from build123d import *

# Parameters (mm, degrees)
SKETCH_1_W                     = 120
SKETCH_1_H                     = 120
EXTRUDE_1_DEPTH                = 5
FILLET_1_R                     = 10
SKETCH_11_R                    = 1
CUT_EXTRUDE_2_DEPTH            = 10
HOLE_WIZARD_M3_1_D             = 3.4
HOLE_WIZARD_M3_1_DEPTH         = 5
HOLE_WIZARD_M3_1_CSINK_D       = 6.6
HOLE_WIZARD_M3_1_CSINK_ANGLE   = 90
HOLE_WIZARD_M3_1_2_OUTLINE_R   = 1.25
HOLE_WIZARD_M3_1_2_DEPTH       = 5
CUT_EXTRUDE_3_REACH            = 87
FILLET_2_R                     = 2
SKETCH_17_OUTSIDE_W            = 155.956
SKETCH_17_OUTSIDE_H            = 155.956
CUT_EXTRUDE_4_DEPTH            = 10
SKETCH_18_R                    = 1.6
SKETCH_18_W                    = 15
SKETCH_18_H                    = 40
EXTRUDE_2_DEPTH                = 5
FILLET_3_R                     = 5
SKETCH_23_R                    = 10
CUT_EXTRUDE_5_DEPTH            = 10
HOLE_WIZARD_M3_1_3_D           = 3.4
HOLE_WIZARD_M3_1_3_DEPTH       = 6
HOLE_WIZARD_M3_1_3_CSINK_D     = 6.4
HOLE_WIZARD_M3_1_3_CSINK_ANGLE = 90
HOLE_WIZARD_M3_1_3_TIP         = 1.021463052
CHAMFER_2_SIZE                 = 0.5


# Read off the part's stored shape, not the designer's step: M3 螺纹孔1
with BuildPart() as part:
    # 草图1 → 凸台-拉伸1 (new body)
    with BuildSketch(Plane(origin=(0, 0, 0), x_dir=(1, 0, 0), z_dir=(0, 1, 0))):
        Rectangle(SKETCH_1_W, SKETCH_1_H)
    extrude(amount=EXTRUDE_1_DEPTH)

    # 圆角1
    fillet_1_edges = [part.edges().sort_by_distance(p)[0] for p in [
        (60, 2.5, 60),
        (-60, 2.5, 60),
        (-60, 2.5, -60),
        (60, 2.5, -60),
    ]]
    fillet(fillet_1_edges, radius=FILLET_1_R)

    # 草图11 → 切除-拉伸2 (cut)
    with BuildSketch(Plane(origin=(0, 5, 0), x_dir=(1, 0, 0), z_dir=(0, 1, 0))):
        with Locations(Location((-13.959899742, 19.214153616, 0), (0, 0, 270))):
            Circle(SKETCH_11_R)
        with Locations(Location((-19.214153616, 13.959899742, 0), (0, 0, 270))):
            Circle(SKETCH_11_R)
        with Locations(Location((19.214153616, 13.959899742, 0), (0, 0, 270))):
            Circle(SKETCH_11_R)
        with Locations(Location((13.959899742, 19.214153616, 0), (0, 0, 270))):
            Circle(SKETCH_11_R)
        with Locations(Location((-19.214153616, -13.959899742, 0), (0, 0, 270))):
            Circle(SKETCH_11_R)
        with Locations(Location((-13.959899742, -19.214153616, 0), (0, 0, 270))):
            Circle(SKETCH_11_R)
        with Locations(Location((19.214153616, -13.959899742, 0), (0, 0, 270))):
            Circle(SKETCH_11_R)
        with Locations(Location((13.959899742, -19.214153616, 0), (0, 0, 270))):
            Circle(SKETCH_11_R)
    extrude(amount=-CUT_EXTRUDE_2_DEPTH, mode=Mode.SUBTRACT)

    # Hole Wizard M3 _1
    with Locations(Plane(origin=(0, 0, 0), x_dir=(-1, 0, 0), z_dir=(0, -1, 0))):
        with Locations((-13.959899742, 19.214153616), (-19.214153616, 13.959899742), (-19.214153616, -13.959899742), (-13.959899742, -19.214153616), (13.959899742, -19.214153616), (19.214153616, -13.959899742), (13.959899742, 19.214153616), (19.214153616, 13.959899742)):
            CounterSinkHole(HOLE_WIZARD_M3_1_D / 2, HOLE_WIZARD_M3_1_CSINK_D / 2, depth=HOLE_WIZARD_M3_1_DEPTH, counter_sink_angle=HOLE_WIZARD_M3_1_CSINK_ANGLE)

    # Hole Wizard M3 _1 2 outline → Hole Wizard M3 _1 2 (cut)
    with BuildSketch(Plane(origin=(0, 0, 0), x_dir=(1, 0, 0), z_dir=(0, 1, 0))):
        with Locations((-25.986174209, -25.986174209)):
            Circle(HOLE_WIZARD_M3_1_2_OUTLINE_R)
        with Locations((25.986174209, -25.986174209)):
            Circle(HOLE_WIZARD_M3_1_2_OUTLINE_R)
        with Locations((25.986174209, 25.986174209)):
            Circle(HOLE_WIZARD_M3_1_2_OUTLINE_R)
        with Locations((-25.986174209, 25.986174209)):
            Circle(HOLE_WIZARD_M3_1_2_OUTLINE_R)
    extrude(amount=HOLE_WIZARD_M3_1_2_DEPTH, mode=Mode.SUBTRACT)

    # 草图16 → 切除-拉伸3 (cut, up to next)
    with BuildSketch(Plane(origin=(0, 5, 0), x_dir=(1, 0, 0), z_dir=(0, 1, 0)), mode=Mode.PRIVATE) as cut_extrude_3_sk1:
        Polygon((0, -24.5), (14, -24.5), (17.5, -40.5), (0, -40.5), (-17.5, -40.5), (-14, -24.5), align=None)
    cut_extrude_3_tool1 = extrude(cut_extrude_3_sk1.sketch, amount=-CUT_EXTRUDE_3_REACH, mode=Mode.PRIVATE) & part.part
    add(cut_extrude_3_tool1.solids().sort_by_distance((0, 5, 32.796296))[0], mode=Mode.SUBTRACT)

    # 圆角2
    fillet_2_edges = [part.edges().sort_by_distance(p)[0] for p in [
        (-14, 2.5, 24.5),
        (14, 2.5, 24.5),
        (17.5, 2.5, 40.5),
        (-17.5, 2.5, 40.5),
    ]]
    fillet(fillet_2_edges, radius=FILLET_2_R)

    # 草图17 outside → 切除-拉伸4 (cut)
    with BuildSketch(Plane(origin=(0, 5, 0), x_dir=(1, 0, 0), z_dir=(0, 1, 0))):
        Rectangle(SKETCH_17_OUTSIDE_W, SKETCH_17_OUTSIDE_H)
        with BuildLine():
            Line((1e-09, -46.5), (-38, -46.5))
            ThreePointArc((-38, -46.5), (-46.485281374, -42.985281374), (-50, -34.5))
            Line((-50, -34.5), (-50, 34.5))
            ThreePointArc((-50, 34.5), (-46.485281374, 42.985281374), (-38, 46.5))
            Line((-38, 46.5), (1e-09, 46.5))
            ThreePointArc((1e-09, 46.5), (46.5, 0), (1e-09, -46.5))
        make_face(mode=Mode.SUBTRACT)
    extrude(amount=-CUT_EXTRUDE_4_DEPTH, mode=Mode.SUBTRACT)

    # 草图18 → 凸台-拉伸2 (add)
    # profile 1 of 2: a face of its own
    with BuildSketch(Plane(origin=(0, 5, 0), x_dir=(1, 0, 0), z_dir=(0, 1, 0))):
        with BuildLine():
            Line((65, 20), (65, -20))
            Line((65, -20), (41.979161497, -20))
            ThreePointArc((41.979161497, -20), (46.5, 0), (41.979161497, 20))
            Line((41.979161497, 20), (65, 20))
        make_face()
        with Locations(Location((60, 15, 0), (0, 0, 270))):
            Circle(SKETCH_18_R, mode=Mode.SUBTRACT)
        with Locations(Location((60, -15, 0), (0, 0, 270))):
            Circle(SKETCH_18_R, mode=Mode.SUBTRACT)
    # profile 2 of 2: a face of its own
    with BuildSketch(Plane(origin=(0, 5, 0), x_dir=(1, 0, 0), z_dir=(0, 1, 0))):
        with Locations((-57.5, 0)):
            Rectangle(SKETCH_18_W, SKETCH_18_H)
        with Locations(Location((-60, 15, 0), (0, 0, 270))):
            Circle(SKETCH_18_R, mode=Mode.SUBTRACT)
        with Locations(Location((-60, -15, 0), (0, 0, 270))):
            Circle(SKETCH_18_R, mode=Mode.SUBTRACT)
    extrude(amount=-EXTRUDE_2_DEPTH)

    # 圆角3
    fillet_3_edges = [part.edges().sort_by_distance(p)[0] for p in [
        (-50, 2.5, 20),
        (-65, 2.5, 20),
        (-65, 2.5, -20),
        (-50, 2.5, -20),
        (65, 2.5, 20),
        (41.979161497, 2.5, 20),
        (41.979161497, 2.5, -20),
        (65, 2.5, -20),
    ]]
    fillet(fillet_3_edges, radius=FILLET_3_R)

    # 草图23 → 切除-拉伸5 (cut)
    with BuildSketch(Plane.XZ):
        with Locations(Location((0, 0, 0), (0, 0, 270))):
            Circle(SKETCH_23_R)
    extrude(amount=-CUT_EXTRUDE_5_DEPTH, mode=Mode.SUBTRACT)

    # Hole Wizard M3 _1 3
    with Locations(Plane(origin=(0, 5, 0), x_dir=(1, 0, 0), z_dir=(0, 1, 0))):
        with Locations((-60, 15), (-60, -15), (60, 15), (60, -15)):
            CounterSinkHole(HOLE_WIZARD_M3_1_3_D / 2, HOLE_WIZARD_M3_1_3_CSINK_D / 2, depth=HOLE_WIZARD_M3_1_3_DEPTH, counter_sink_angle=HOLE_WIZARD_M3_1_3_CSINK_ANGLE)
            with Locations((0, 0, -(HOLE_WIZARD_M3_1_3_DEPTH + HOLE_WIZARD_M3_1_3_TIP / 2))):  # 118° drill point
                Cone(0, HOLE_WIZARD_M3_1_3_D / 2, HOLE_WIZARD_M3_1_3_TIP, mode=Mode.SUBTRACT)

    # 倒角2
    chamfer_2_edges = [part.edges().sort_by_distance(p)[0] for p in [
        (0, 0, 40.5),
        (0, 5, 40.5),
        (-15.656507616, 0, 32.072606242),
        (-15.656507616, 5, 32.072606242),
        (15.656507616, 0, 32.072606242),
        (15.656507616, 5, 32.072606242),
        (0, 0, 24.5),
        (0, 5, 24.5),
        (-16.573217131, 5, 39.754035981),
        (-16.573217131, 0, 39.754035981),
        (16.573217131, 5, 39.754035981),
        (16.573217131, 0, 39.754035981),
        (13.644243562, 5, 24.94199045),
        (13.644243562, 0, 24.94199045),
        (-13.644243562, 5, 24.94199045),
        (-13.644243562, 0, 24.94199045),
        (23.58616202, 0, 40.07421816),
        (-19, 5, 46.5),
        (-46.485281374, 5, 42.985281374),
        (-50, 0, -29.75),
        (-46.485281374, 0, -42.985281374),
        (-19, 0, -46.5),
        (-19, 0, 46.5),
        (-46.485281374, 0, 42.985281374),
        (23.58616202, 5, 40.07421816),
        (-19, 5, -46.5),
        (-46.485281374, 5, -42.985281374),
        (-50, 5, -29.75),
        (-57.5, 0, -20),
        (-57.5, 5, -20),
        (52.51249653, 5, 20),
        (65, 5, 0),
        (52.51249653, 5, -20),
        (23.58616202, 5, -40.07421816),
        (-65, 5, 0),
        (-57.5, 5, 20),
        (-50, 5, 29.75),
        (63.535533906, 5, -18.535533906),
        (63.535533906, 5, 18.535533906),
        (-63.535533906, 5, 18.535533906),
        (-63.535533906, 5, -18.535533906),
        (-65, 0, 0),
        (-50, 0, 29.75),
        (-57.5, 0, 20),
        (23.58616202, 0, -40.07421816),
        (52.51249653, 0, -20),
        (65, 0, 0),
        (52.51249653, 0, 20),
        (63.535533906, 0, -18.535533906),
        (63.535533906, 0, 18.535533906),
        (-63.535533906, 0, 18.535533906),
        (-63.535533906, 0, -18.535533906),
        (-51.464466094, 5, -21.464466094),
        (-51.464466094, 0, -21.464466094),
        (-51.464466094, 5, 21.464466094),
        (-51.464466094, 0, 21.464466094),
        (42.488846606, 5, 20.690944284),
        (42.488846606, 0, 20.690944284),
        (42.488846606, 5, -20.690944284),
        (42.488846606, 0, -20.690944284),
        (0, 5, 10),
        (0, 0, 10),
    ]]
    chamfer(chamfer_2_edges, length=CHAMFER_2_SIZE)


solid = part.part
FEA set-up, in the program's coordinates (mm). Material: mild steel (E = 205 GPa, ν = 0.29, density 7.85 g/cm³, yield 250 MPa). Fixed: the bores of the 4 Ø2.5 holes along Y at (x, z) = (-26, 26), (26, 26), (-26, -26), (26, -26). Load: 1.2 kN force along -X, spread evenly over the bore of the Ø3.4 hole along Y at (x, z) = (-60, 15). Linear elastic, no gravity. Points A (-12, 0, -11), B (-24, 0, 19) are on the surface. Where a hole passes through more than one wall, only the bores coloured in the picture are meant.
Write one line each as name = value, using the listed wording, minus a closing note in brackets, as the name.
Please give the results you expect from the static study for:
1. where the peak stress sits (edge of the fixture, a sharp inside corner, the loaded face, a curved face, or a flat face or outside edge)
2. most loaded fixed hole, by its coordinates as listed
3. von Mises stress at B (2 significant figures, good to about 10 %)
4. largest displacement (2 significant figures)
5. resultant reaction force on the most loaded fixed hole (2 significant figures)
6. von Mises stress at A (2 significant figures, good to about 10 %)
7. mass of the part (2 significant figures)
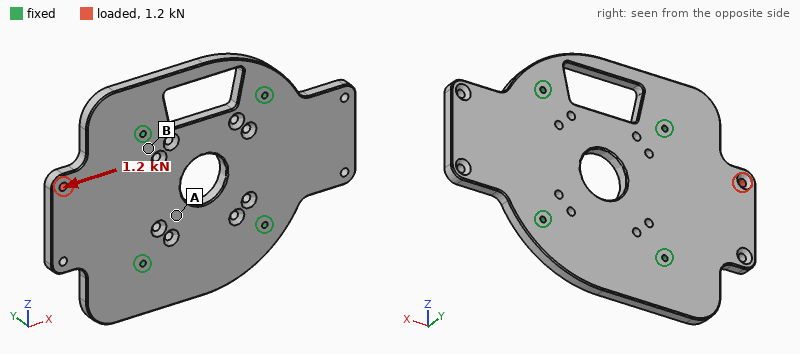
where the peak stress sits = the loaded face
most loaded fixed hole, by its coordinates as listed = (-26, 26)
von Mises stress at B = 6.6 MPa
largest displacement = 9.4 µm
resultant reaction force on the most loaded fixed hole = 780 N
von Mises stress at A = 3.6 MPa
mass of the part = 330 g
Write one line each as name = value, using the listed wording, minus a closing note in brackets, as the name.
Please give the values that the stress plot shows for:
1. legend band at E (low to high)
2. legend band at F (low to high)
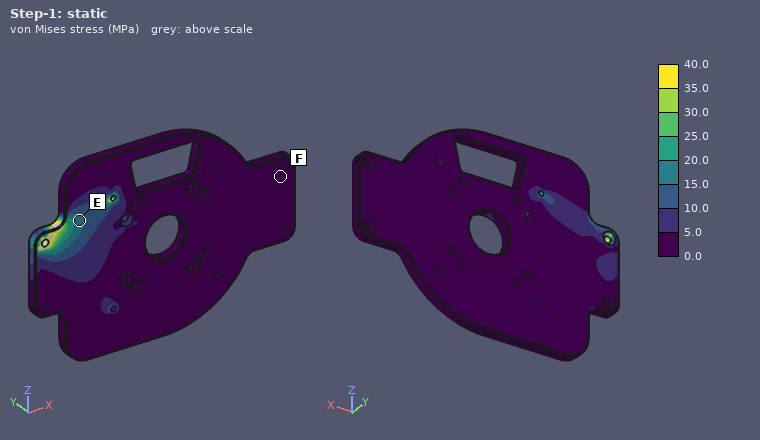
legend band at E = 15.0 to 20.0 MPa
legend band at F = 0.0 to 5.0 MPa
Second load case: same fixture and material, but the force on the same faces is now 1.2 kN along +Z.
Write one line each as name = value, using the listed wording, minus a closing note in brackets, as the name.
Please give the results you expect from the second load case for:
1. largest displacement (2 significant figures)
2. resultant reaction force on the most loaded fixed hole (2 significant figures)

largest displacement = 5.9 µm
resultant reaction force on the most loaded fixed hole = 870 N
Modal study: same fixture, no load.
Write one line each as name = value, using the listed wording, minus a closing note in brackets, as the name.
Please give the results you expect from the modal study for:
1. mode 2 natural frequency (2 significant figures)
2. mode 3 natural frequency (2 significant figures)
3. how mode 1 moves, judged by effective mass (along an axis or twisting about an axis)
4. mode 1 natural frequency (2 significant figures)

mode 2 natural frequency = 2700 Hz
mode 3 natural frequency = 5600 Hz
how mode 1 moves, judged by effective mass = along Y
mode 1 natural frequency = 2400 Hz
